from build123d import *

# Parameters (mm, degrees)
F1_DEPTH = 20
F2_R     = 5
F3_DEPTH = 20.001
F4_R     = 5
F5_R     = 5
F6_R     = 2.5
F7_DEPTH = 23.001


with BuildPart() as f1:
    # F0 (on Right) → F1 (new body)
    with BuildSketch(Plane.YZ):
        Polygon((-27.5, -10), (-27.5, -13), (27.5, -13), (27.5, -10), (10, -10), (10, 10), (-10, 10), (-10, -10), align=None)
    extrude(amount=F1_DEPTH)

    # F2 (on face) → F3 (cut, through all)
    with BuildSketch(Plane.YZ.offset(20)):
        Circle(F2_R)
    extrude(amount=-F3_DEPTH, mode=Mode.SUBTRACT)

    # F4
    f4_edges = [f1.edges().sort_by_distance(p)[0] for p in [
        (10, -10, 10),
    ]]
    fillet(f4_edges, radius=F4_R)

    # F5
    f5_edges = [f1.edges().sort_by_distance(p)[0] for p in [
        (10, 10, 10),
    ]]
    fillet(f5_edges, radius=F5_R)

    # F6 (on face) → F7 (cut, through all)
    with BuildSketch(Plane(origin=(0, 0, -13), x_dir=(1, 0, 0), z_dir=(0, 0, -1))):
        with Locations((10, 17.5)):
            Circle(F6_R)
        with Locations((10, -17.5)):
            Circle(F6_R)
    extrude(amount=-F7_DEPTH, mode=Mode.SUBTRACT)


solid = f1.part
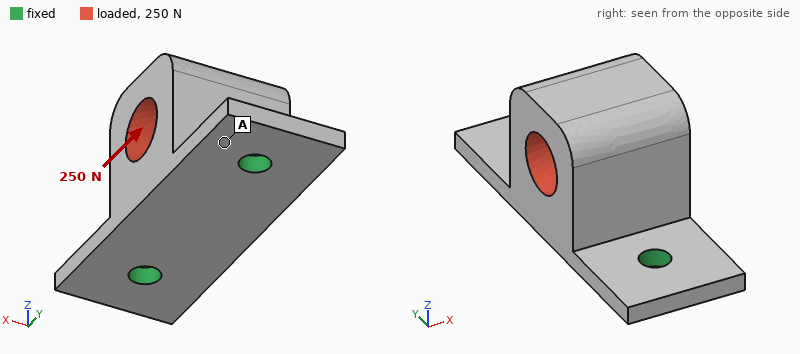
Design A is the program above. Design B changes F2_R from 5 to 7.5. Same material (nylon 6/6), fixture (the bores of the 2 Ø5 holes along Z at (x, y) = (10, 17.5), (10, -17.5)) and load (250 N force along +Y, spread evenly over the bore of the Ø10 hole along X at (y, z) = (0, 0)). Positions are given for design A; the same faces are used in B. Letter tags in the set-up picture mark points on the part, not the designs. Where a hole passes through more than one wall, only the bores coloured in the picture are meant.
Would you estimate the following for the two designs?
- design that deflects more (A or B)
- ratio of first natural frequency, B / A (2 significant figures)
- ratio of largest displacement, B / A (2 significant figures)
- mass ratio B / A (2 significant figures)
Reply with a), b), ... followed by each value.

a) B
b) 1.2
c) 1.5
d) 0.79
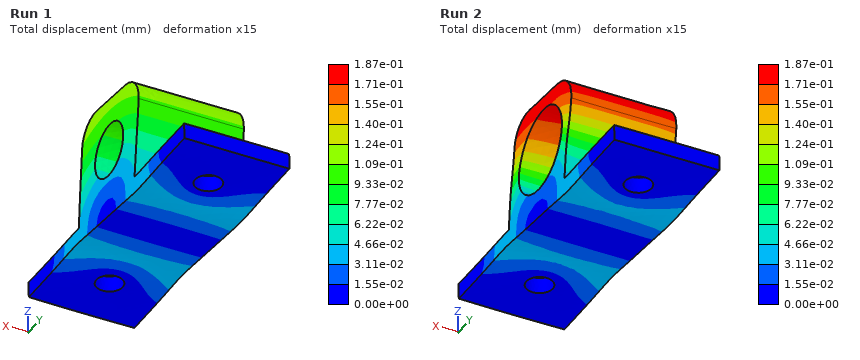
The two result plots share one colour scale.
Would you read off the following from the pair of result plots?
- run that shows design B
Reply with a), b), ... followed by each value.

a) Run 2
